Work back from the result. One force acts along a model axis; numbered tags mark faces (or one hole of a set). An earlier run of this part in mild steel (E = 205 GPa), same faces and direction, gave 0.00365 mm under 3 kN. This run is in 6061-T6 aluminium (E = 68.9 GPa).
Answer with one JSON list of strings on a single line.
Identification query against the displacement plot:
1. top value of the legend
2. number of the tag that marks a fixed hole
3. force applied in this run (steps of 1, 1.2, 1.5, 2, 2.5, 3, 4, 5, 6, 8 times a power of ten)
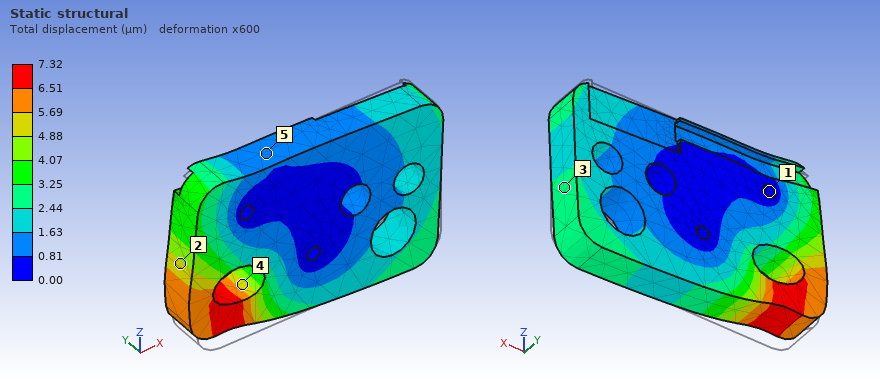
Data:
["7.32 µm", "1", "2 kN"]
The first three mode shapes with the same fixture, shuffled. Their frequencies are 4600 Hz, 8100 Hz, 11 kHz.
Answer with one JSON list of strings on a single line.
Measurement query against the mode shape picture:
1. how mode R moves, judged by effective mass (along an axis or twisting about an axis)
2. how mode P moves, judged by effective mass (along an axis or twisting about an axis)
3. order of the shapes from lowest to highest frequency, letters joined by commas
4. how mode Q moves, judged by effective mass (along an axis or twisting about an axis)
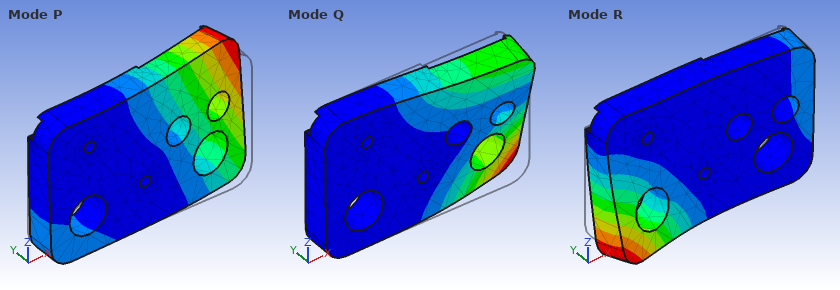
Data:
["along Y", "along Y", "P, Q, R", "twisting about X"]
